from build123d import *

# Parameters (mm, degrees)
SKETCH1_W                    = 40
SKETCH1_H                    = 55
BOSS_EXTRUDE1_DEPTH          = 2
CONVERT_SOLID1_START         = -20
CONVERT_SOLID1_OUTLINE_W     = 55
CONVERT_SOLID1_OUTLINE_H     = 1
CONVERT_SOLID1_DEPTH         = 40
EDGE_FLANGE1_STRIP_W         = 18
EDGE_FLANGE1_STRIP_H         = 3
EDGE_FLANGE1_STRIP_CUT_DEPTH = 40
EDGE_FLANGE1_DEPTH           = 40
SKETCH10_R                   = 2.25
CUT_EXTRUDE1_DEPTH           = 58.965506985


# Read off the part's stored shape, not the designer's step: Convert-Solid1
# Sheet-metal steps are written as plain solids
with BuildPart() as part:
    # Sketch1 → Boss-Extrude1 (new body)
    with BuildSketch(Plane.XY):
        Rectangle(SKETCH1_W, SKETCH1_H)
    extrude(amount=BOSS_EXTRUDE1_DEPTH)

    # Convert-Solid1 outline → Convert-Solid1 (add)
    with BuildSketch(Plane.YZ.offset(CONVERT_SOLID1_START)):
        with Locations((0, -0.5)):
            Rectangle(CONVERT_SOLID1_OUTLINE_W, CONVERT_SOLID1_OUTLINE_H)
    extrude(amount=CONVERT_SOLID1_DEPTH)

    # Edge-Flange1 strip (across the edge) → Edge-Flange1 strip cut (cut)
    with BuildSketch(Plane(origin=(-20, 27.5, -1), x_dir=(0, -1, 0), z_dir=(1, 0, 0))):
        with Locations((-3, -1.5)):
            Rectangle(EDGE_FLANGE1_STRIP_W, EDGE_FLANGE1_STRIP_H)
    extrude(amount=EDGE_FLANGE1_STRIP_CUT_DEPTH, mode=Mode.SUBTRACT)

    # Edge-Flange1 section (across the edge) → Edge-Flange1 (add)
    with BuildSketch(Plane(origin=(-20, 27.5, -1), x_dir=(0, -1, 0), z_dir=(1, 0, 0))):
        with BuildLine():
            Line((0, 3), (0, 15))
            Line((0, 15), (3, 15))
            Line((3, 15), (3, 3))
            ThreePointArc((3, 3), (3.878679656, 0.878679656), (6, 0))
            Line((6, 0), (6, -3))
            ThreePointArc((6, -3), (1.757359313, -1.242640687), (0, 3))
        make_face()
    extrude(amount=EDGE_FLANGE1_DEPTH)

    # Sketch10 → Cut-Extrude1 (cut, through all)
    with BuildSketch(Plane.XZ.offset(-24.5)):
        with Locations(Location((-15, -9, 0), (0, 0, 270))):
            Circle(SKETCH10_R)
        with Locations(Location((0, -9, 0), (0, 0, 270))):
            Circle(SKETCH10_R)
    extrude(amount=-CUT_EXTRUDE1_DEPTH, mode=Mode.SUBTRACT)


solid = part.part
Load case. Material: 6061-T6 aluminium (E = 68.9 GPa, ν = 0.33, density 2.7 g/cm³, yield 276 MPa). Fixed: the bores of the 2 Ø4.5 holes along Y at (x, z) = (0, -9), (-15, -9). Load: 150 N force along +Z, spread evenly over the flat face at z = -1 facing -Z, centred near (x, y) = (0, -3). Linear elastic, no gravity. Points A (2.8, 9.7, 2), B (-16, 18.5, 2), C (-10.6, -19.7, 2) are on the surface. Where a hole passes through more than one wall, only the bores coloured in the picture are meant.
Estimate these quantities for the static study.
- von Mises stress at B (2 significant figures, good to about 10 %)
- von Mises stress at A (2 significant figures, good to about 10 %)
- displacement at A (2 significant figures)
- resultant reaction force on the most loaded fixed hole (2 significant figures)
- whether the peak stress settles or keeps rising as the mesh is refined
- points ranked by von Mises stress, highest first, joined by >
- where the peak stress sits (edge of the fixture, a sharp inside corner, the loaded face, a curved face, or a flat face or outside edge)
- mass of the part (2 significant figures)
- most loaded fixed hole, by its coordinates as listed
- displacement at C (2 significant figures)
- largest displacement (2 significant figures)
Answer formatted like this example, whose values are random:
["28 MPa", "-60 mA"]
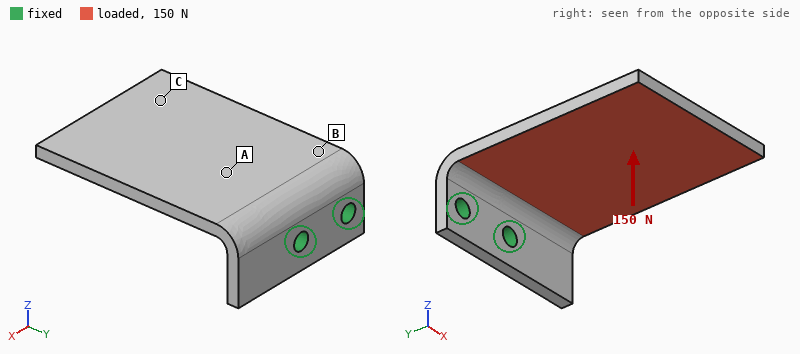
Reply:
["56 MPa", "31 MPa", "0.17 mm", "130 N", "keeps rising", "B > A > C", "edge of the fixture", "22 g", "(0, -9)", "0.63 mm", "0.78 mm"]
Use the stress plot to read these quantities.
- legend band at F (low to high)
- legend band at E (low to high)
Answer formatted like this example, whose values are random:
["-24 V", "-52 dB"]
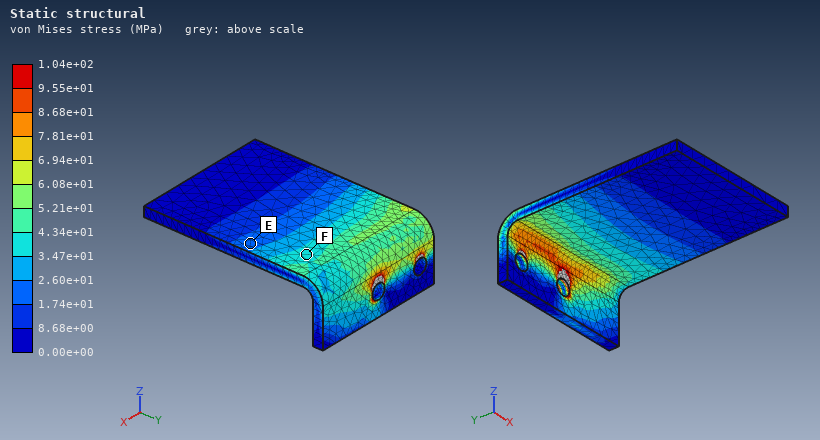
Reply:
["3.47e+01 to 4.34e+01 MPa", "1.74e+01 to 2.60e+01 MPa"]
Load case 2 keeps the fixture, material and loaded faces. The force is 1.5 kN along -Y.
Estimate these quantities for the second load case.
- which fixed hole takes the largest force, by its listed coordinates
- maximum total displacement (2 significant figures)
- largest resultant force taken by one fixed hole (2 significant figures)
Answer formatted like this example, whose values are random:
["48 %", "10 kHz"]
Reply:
["(0, -9)", "0.26 mm", "1.3 kN"]
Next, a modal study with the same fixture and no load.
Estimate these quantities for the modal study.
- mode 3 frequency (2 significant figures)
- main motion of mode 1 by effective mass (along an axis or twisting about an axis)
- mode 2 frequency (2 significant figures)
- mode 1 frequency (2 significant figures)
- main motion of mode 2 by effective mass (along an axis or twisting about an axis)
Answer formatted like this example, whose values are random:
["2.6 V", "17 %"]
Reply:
["2600 Hz", "along Z", "1900 Hz", "690 Hz", "along X"]
